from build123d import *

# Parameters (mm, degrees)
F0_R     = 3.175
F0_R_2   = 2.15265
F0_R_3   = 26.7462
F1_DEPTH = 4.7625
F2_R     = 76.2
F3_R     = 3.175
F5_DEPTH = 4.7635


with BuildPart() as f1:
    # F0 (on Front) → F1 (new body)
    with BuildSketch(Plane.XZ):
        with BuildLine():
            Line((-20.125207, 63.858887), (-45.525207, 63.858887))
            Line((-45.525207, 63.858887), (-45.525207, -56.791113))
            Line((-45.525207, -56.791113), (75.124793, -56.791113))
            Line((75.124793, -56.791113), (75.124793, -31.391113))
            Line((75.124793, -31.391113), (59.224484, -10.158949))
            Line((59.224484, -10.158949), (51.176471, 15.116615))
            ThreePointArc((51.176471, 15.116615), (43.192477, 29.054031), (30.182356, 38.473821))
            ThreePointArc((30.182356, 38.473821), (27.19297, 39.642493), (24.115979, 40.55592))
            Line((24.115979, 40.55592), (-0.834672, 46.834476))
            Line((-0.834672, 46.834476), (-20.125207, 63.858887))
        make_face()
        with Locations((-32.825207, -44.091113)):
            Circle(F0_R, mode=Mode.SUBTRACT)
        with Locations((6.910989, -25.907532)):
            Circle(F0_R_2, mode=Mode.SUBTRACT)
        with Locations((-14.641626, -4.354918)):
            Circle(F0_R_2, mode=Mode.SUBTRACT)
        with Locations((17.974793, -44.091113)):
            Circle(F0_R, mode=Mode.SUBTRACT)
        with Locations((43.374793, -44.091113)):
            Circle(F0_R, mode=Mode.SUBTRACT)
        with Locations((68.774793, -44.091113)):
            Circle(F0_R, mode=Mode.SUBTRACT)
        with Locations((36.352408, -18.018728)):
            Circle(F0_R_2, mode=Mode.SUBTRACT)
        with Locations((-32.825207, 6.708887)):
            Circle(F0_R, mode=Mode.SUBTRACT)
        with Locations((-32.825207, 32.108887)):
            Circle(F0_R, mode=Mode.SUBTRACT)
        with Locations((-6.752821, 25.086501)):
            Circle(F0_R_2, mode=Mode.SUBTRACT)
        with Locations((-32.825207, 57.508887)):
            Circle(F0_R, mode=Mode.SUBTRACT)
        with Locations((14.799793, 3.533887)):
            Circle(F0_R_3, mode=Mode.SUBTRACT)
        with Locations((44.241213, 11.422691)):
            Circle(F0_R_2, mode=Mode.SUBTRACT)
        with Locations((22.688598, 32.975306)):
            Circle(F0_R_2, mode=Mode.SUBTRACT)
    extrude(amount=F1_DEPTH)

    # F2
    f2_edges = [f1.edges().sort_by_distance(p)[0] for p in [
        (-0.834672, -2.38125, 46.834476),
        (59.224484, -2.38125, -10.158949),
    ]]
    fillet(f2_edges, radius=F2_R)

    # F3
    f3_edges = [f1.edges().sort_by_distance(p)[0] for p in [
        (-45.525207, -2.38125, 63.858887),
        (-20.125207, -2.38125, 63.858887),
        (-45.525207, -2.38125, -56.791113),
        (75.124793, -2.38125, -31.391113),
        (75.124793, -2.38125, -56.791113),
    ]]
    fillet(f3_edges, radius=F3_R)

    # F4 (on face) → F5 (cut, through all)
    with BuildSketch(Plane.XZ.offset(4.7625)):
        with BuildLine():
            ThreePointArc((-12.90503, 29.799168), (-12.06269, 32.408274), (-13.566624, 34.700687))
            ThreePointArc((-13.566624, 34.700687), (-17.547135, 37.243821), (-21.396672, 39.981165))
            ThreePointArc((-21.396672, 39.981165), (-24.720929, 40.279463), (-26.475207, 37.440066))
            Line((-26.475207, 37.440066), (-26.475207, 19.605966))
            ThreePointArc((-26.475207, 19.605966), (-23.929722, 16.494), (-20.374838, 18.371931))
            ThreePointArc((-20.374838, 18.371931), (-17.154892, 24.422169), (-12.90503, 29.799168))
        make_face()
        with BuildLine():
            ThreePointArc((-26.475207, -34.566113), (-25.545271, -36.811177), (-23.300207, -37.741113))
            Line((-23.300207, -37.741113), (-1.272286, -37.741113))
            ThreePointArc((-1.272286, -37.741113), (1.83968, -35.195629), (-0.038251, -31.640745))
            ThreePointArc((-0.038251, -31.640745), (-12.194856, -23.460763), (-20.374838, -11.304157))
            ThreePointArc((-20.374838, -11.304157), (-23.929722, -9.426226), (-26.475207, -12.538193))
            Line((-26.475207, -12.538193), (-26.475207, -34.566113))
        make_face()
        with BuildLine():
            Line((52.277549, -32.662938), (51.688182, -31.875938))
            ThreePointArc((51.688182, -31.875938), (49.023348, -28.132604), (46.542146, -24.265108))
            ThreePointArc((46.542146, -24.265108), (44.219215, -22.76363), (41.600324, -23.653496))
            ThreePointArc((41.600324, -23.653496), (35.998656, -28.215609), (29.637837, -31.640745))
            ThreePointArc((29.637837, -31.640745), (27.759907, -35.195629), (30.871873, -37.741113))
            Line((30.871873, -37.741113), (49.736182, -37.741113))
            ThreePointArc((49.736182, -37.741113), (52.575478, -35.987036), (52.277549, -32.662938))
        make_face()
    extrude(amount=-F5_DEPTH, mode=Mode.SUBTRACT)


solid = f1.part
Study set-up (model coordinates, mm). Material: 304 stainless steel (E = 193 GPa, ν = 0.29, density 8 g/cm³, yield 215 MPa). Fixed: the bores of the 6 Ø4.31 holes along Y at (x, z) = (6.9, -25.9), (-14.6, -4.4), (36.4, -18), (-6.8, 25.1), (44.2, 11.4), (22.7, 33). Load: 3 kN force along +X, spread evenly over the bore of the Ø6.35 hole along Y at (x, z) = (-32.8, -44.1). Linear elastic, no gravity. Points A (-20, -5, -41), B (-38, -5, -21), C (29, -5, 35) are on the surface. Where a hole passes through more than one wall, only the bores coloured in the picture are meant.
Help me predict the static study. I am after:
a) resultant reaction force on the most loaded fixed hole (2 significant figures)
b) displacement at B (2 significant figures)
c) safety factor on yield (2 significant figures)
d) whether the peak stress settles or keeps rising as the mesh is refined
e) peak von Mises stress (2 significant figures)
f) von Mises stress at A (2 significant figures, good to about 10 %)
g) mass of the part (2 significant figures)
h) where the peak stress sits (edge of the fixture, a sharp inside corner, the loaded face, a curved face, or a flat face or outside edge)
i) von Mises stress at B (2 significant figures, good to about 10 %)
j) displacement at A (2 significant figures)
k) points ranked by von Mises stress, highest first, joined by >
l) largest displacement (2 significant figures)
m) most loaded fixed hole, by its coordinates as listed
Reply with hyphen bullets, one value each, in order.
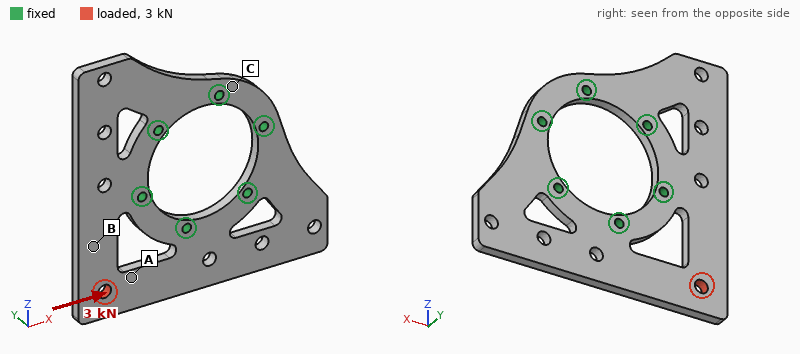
- 1.7 kN
- 7.4 µm
- 2.2
- settles
- 99 MPa
- 32 MPa
- 290 g
- a curved face
- 13 MPa
- 11 µm
- A > B > C
- 15 µm
- (6.9, -25.9)
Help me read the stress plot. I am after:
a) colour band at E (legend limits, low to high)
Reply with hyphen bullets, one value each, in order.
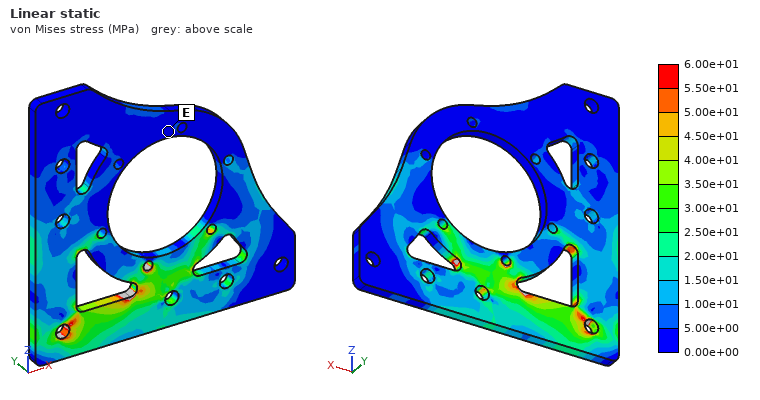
- 0.00e+00 to 5.00e+00 MPa
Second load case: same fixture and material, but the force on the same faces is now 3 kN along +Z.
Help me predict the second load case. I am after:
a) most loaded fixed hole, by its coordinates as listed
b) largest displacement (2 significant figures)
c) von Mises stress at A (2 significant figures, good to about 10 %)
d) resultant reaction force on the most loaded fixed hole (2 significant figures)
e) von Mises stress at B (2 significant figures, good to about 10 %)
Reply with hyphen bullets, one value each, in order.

- (-14.6, -4.4)
- 15 µm
- 16 MPa
- 1.7 kN
- 24 MPa
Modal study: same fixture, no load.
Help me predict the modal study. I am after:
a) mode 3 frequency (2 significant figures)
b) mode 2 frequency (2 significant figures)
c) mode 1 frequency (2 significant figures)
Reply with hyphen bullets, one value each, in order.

- 1500 Hz
- 1500 Hz
- 1400 Hz
